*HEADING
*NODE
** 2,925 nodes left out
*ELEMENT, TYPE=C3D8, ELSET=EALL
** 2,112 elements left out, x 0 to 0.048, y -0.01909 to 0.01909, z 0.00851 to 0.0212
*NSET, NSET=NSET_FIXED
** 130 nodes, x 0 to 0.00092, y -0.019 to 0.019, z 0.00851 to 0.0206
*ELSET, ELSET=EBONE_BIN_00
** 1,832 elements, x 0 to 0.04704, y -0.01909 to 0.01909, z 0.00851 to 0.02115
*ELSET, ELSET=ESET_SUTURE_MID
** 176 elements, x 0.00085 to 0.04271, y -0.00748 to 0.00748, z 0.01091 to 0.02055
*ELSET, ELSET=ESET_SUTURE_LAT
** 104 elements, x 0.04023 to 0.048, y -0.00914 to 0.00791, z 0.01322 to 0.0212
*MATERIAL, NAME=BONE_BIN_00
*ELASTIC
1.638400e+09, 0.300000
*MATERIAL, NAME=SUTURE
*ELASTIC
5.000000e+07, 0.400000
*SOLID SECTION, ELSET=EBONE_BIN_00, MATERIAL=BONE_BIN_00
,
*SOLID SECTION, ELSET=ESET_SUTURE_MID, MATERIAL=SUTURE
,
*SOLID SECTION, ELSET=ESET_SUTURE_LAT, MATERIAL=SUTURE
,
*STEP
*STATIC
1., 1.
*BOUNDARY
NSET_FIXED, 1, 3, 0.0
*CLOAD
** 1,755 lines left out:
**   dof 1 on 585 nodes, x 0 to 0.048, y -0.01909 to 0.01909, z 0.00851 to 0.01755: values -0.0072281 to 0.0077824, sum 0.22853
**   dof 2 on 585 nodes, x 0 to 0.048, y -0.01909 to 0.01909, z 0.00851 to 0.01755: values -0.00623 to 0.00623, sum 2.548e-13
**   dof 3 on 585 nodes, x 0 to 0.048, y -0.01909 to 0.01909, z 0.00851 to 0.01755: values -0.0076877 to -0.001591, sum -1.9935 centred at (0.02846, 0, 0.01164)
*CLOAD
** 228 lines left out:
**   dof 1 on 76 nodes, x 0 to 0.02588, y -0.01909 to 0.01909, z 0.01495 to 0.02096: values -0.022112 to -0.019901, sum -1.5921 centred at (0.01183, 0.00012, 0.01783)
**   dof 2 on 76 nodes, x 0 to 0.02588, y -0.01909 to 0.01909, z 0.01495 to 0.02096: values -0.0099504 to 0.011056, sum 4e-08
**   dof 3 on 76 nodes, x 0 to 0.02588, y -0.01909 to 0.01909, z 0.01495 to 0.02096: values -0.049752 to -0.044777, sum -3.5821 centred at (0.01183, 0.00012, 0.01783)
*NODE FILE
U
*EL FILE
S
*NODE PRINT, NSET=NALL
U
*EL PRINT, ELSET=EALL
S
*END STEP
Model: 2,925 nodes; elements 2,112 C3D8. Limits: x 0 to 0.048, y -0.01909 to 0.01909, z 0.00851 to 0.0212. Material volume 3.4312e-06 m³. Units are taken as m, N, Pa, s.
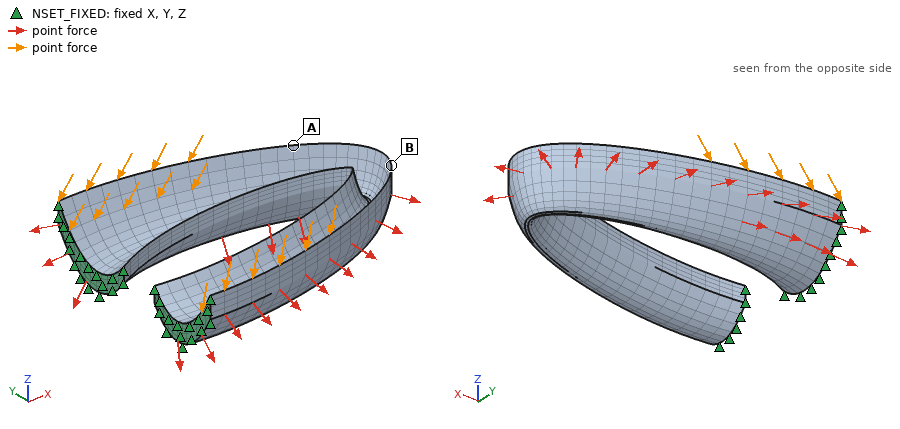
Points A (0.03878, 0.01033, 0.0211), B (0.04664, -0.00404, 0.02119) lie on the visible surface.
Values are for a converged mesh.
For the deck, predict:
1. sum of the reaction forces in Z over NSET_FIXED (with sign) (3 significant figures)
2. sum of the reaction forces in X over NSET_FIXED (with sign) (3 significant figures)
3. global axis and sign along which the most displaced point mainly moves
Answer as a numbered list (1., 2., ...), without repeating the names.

1. 5.58 N
2. 1.36 N
3. -Z
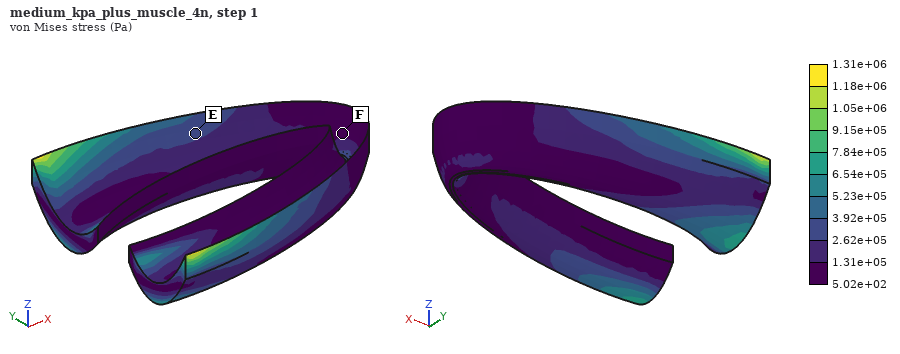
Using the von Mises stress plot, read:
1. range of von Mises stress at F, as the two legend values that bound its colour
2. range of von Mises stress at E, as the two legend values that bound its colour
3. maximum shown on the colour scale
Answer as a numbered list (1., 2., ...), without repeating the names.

1. 5.02e+02 to 1.31e+05 Pa
2. 2.62e+05 to 3.92e+05 Pa
3. 1.31e+06 Pa
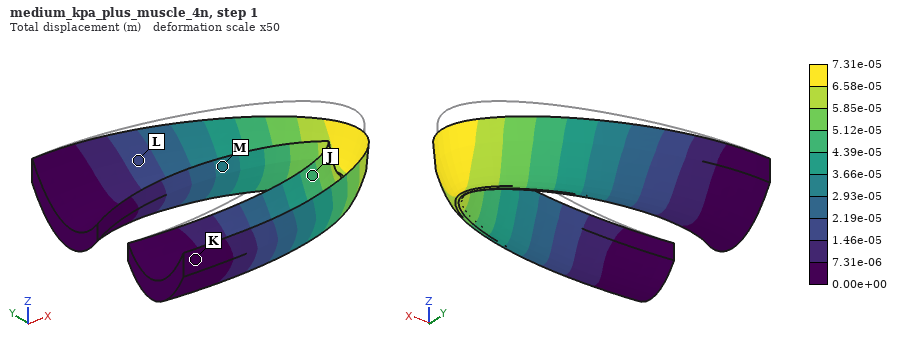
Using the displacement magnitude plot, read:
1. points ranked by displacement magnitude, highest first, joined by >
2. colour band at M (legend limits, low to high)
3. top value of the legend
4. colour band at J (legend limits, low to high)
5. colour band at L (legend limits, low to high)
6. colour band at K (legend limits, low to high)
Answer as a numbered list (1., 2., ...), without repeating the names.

1. J > M > L > K
2. 2.93e-05 to 3.66e-05 m
3. 7.31e-05 m
4. 4.39e-05 to 5.12e-05 m
5. 1.46e-05 to 2.19e-05 m
6. 0.00e+00 to 7.31e-06 m
